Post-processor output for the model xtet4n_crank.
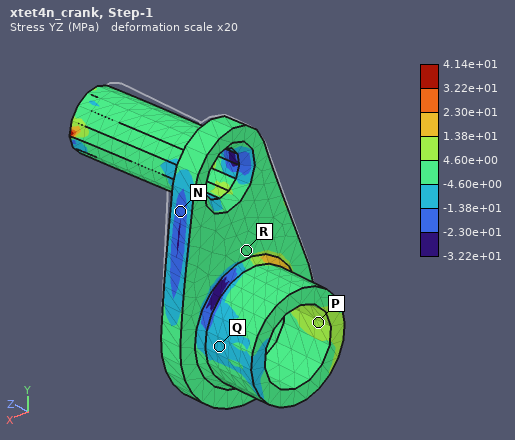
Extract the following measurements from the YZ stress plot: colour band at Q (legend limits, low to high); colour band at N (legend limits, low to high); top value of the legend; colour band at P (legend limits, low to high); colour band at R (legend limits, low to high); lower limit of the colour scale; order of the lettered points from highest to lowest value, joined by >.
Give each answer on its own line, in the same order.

-1.38e+01 to -4.60e+00 MPa
-2.30e+01 to -1.38e+01 MPa
4.14e+01 MPa
4.60e+00 to 1.38e+01 MPa
-4.60e+00 to 4.60e+00 MPa
-3.22e+01 MPa
P > R > Q > N
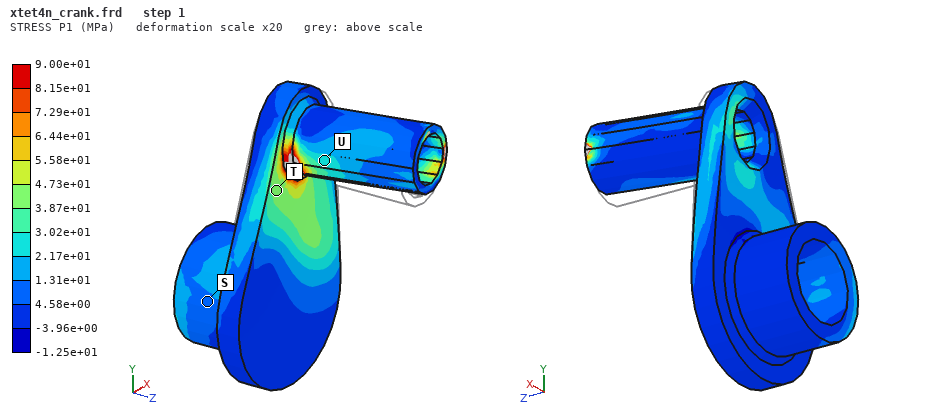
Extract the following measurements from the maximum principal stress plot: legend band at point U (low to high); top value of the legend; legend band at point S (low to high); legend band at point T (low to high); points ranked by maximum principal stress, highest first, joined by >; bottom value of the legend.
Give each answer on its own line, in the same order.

2.17e+01 to 3.02e+01 MPa
9.00e+01 MPa
4.58e+00 to 1.31e+01 MPa
3.87e+01 to 4.73e+01 MPa
T > U > S
-1.25e+01 MPa
